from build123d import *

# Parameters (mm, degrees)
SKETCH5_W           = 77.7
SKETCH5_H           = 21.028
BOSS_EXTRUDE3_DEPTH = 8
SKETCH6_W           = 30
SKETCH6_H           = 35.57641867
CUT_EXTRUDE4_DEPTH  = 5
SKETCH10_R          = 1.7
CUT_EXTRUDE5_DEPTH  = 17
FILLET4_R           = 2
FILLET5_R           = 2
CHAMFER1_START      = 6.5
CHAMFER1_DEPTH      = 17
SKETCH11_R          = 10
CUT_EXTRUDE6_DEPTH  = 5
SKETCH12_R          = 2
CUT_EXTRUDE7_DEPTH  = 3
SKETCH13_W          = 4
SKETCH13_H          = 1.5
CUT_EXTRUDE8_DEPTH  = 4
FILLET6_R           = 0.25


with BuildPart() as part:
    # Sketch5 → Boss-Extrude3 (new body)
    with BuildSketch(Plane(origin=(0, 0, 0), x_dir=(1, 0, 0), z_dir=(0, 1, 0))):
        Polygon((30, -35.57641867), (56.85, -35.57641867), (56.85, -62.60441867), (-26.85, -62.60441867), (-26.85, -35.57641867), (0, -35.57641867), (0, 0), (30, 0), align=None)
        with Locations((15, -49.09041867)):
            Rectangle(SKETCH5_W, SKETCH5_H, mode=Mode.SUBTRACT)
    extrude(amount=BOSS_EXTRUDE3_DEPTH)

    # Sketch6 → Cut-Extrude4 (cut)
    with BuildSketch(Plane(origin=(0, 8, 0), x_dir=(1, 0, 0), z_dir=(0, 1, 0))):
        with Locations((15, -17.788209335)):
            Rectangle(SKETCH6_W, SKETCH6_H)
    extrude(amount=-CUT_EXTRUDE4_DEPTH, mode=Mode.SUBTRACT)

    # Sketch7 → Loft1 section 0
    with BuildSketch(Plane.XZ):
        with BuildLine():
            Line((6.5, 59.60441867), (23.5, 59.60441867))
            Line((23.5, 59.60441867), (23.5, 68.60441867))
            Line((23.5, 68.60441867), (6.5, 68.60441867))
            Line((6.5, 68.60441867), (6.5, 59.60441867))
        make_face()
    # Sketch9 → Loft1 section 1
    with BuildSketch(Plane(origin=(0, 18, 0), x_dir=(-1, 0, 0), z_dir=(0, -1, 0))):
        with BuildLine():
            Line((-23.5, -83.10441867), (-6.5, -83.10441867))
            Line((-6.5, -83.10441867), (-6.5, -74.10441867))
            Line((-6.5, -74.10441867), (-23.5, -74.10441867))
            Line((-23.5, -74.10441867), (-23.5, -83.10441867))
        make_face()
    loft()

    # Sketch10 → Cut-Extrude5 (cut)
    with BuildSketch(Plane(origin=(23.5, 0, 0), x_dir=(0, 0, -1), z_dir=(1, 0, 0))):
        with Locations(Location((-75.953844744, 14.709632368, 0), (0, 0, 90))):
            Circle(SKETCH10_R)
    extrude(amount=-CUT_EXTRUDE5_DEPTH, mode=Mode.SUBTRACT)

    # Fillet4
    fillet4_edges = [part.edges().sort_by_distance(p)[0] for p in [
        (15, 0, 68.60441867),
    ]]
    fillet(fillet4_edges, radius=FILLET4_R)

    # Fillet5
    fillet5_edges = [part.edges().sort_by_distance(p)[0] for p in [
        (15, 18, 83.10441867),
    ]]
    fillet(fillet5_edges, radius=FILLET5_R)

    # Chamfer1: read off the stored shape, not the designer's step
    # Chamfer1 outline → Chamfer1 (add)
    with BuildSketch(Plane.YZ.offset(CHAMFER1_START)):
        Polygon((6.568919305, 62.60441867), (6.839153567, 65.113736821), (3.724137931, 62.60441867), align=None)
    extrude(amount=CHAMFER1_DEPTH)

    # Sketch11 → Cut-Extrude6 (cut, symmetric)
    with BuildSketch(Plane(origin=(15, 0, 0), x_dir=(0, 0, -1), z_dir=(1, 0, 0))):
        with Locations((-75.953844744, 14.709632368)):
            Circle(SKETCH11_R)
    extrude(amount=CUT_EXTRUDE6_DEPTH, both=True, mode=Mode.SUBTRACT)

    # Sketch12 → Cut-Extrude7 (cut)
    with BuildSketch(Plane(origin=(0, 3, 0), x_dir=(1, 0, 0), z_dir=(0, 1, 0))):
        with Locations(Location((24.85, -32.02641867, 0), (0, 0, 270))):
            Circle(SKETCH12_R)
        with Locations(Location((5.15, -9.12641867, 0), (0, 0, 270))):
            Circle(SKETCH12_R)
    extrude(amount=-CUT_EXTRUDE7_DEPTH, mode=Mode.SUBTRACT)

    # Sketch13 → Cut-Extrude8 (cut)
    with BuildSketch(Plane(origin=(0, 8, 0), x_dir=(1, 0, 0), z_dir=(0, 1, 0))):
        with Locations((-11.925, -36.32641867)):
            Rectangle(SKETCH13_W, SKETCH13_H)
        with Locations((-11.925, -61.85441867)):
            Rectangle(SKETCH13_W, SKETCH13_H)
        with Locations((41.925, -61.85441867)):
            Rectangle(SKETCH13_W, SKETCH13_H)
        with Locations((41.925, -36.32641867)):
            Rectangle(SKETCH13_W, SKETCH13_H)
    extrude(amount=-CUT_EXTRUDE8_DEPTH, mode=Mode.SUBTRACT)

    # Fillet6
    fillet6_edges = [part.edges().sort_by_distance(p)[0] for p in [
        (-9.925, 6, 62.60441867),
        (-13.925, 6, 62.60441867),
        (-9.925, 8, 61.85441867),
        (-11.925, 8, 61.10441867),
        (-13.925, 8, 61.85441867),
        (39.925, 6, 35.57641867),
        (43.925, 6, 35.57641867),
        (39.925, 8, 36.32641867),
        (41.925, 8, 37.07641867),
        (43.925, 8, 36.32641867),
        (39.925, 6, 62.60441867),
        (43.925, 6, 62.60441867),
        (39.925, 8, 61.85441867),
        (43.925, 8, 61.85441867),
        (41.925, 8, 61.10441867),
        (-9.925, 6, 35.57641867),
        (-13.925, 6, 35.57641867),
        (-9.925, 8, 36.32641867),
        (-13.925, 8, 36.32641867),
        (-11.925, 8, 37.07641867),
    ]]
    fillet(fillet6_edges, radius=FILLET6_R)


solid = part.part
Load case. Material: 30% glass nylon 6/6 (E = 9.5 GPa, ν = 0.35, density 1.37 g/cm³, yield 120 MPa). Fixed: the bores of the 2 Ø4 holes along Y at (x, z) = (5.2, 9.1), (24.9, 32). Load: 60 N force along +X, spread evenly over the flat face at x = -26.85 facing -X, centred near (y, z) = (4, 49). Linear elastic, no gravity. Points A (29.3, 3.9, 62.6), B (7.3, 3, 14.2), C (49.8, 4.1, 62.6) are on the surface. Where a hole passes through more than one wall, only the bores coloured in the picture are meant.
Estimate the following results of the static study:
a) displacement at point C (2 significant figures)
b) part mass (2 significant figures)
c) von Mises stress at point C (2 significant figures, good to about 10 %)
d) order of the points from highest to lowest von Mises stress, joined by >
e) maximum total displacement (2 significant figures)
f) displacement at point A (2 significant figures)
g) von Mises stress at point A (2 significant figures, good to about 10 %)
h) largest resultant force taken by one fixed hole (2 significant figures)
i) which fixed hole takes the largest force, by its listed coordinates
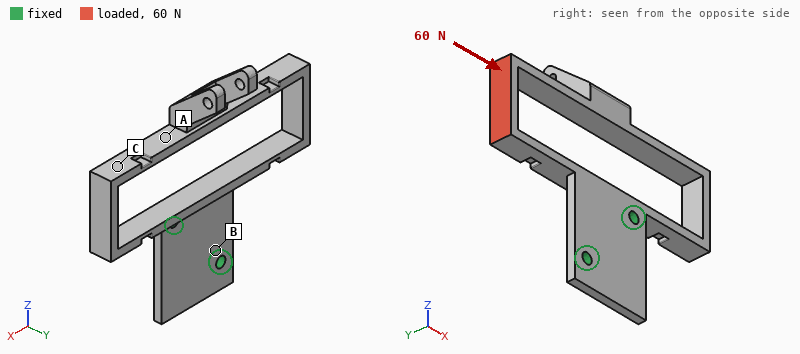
1.2 mm
13 g
14 MPa
C > A > B
1.3 mm
1.0 mm
6.3 MPa
76 N
(24.9, 32)
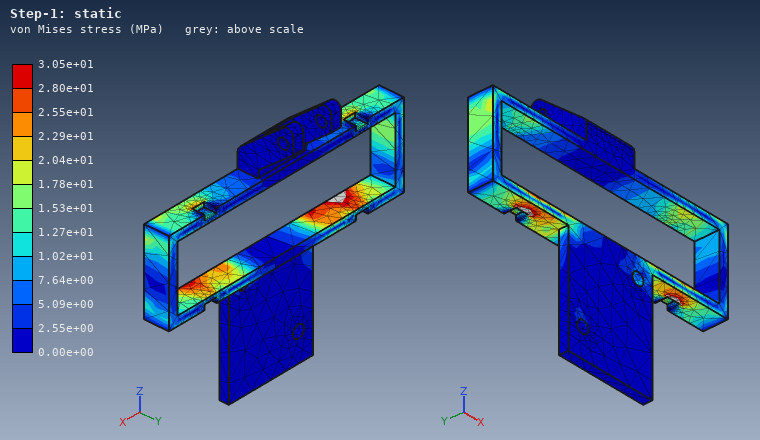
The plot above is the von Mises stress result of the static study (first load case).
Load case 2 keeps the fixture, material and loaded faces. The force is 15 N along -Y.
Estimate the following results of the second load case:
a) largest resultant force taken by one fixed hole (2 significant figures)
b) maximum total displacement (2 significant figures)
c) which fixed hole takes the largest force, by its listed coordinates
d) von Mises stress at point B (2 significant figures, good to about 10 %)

14 N
1.2 mm
(24.9, 32)
5.6 MPa
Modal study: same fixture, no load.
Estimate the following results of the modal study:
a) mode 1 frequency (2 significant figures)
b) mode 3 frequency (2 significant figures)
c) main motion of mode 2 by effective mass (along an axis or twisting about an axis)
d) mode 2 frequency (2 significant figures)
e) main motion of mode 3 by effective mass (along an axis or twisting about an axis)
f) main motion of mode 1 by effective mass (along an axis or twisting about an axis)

230 Hz
470 Hz
along X
330 Hz
along Z
along Y
